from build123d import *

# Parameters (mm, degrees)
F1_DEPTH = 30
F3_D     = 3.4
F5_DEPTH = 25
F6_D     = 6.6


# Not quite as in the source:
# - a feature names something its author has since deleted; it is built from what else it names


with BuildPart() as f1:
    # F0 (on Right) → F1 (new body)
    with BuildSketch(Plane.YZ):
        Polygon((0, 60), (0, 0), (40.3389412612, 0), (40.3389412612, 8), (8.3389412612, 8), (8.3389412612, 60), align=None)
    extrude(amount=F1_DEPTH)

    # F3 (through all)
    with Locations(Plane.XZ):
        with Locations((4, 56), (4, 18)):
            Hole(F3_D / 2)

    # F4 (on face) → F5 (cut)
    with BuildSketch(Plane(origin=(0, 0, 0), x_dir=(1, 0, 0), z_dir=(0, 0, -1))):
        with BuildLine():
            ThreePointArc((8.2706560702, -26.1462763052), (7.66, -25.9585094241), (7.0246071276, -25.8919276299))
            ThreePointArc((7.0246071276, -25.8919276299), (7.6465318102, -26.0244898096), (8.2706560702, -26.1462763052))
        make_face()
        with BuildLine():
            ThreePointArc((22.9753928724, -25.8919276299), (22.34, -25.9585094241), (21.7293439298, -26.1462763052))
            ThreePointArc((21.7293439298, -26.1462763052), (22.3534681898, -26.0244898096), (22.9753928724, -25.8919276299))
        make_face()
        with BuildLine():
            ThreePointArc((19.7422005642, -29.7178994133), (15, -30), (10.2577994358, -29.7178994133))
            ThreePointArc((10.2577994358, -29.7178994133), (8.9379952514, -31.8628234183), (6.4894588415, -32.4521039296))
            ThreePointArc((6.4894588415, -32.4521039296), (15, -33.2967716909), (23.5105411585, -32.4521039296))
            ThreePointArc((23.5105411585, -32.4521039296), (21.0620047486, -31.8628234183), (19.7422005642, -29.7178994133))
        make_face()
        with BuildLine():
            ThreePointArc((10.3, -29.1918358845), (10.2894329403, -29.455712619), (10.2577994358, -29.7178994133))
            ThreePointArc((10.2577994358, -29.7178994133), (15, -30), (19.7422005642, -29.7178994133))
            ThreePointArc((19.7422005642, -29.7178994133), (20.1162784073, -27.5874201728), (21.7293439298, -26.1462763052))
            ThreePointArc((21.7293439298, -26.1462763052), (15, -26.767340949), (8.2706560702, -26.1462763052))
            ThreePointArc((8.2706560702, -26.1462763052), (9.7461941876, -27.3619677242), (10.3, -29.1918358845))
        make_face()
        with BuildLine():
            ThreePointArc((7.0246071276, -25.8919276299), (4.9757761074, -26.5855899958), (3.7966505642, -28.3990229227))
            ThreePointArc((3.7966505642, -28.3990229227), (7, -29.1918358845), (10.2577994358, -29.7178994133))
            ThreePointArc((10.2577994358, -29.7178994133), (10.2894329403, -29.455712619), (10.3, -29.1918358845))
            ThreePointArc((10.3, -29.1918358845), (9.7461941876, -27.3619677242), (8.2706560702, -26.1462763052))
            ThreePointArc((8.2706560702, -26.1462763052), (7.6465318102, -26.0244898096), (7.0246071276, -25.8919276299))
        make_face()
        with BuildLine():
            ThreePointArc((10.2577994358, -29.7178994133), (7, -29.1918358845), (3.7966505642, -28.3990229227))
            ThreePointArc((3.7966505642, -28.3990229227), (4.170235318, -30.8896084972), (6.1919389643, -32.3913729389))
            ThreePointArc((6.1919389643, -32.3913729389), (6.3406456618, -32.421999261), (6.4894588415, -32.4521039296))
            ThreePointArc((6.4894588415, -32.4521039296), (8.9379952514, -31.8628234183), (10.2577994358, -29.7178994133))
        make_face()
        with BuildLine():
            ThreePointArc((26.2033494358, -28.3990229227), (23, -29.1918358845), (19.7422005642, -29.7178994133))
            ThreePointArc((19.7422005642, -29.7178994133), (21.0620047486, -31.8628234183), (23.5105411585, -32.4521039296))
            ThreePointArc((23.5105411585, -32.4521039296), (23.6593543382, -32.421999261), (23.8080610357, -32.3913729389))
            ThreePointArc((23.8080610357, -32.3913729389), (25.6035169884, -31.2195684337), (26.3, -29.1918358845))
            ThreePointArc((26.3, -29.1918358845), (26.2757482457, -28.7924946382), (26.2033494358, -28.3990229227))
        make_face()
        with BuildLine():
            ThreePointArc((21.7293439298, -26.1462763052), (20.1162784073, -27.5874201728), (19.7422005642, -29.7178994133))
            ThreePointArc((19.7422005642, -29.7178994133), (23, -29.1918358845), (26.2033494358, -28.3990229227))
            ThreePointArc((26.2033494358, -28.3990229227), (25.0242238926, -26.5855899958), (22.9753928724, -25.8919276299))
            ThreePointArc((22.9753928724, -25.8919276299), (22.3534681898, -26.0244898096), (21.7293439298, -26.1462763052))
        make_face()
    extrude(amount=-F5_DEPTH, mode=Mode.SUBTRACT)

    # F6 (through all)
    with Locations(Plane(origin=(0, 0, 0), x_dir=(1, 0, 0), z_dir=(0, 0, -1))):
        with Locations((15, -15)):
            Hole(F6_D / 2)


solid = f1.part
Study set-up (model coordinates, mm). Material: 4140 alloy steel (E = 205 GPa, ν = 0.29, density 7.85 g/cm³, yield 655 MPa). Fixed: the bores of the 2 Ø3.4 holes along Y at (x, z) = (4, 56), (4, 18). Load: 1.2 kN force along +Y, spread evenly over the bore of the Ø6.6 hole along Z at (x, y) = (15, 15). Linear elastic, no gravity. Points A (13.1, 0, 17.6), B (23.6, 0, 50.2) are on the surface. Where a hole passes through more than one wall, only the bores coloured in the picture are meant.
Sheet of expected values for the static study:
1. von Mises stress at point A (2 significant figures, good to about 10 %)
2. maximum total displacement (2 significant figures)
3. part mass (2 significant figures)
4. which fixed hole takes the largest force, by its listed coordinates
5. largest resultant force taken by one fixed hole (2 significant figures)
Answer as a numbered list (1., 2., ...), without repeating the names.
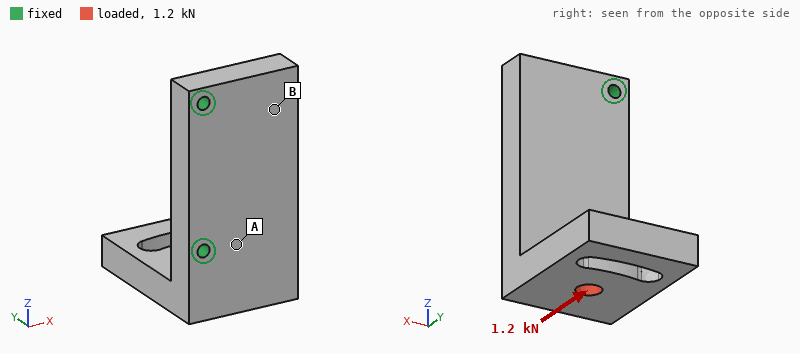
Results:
1. 34 MPa
2. 41 µm
3. 170 g
4. (4, 18)
5. 1.4 kN
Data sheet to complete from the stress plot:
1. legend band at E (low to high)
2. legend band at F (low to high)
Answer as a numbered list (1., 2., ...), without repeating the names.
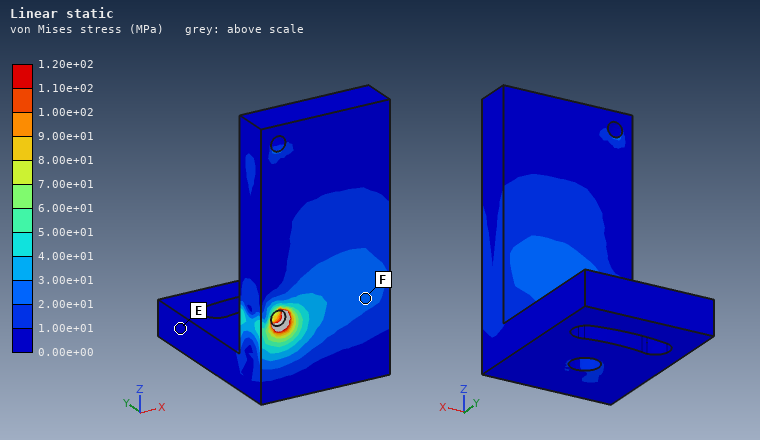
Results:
1. 0.00e+00 to 1.00e+01 MPa
2. 2.00e+01 to 3.00e+01 MPa
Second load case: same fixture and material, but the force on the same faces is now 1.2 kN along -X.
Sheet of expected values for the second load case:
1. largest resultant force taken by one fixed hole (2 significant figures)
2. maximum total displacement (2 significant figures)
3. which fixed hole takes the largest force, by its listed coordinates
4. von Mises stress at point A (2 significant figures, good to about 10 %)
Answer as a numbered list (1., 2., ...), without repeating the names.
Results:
1. 1.6 kN
2. 33 µm
3. (4, 18)
4. 18 MPa
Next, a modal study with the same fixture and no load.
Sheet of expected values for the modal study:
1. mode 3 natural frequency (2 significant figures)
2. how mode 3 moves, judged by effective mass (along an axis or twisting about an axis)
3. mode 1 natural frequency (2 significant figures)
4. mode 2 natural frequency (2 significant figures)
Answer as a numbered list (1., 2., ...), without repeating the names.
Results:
1. 8500 Hz
2. along Y
3. 3000 Hz
4. 3500 Hz
